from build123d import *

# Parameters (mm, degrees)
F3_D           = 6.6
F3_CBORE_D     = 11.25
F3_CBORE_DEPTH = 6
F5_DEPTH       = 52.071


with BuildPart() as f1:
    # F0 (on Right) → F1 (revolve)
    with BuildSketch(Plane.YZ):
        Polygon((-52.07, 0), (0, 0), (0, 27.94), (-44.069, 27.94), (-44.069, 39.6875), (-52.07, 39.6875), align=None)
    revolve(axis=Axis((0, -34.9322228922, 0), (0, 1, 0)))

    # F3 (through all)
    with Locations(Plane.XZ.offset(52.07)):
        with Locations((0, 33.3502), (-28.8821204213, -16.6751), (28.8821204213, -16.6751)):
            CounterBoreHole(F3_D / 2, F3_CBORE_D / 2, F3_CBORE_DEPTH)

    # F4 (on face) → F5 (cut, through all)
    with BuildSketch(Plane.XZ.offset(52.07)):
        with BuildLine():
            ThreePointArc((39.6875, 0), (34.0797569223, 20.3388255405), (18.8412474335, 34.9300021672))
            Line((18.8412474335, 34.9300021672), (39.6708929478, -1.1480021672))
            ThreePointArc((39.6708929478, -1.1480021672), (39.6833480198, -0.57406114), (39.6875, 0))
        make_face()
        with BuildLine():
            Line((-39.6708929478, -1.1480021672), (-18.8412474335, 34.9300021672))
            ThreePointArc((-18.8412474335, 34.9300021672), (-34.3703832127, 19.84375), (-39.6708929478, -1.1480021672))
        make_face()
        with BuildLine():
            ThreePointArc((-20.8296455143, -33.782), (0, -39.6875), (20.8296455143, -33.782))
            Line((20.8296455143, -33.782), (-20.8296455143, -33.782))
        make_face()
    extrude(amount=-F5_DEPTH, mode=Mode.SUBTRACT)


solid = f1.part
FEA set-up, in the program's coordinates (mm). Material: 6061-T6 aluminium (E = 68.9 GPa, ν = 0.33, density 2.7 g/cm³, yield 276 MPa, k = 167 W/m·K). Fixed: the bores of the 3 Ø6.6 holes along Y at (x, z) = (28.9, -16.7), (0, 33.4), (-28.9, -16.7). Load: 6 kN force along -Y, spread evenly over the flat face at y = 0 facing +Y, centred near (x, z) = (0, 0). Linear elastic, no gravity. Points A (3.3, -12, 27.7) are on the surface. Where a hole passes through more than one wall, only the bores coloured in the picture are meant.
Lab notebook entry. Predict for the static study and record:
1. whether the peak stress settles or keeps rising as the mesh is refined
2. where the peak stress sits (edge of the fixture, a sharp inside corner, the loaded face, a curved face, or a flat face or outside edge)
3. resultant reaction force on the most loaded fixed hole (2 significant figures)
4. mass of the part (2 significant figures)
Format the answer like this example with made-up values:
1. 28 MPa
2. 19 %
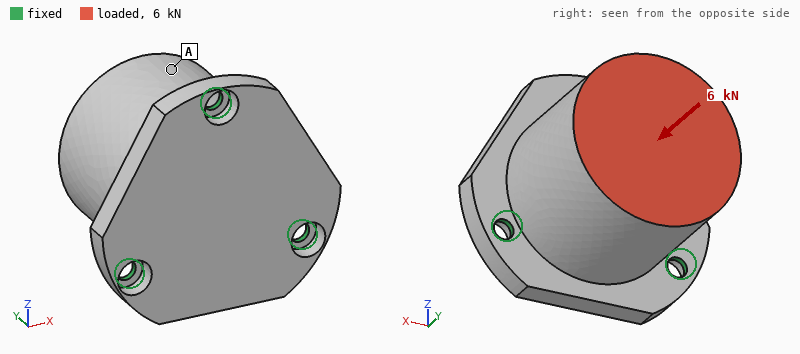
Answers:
1. keeps rising
2. edge of the fixture
3. 2.0 kN
4. 380 g
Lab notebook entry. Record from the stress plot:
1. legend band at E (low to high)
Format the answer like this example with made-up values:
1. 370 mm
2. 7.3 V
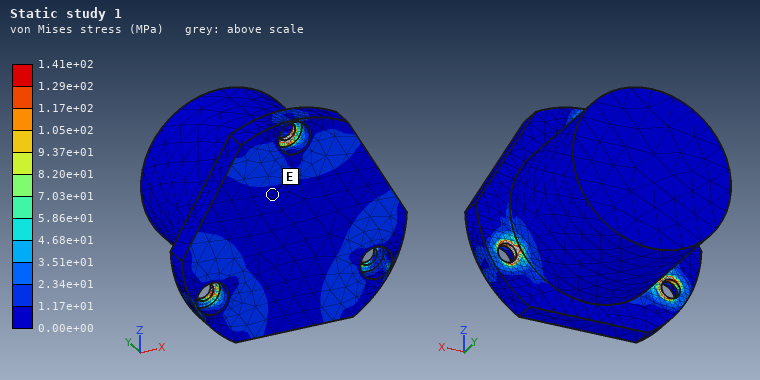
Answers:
1. 0.00e+00 to 1.17e+01 MPa
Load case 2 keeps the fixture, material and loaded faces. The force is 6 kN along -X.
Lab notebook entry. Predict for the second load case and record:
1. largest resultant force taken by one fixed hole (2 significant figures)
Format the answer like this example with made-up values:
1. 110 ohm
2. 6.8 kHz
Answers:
1. 5.2 kN
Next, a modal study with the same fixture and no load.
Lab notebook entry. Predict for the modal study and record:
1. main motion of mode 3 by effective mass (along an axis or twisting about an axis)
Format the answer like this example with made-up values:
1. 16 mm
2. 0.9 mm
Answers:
1. along Y
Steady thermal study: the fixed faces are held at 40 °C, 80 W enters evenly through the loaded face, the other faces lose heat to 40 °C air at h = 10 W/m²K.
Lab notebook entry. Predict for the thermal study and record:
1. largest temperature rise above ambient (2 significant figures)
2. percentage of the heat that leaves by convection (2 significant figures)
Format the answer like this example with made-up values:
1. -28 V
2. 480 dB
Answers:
1. 24 K
2. 3.3 %
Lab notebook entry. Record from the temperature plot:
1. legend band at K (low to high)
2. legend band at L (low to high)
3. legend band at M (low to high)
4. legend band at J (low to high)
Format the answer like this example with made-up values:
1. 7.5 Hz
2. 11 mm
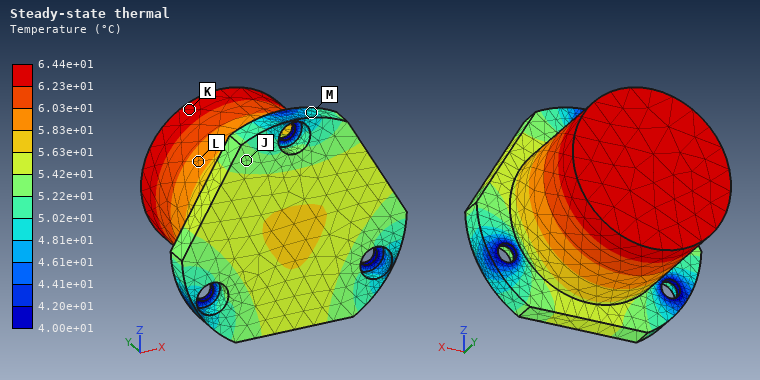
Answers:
1. 6.23e+01 to 6.44e+01 °C
2. 5.83e+01 to 6.03e+01 °C
3. 4.81e+01 to 5.02e+01 °C
4. 5.22e+01 to 5.42e+01 °C
